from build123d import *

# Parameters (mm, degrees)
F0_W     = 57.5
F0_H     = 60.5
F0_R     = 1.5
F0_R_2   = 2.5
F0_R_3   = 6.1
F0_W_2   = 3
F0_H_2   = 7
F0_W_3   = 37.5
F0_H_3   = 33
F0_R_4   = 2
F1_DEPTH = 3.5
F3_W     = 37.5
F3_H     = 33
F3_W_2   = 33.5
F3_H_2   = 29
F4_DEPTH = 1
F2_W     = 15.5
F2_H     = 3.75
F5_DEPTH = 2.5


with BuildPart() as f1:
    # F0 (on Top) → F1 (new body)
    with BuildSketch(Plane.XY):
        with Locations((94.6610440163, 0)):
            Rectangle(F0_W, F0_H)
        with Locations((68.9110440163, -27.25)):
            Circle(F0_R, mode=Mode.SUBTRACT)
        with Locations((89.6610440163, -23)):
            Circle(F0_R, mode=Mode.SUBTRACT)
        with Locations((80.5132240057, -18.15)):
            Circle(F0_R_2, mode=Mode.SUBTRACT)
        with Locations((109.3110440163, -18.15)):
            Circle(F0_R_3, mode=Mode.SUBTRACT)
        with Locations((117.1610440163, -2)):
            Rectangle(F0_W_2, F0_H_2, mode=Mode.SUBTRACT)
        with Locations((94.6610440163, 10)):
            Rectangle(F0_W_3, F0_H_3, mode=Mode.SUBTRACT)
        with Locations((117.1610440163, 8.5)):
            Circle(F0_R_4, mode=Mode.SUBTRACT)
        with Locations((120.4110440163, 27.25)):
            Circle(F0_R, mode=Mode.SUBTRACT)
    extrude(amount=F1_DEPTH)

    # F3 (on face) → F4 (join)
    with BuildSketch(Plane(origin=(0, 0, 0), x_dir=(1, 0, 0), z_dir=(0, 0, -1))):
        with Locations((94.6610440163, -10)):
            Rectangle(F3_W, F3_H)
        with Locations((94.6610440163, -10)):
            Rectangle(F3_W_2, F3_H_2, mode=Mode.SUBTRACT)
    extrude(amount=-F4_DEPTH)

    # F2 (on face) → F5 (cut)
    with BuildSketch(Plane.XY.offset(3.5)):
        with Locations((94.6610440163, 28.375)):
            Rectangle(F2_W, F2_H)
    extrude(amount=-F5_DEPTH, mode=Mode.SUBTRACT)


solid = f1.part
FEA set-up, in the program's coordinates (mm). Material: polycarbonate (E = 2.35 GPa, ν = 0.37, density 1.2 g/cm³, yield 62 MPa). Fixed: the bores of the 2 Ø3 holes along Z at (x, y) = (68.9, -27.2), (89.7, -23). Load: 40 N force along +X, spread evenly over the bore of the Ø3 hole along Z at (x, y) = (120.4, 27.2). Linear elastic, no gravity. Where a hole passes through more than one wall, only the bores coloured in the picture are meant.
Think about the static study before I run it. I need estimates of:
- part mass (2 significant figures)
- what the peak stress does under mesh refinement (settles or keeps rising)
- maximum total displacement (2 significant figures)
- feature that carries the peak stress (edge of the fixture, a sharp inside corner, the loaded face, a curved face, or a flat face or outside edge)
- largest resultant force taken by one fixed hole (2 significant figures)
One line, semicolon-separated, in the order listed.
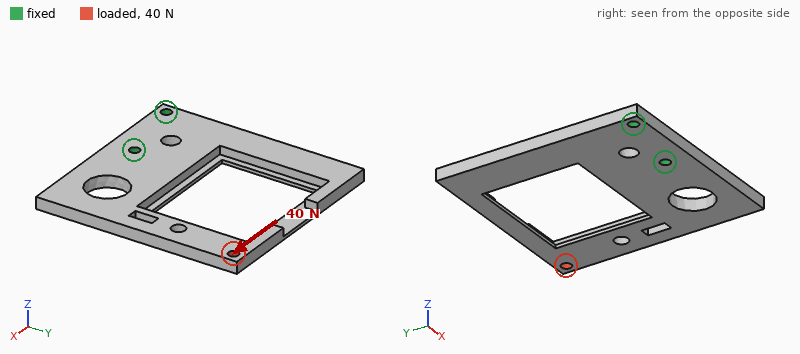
8.8 g; keeps rising; 0.85 mm; a sharp inside corner; 95 N
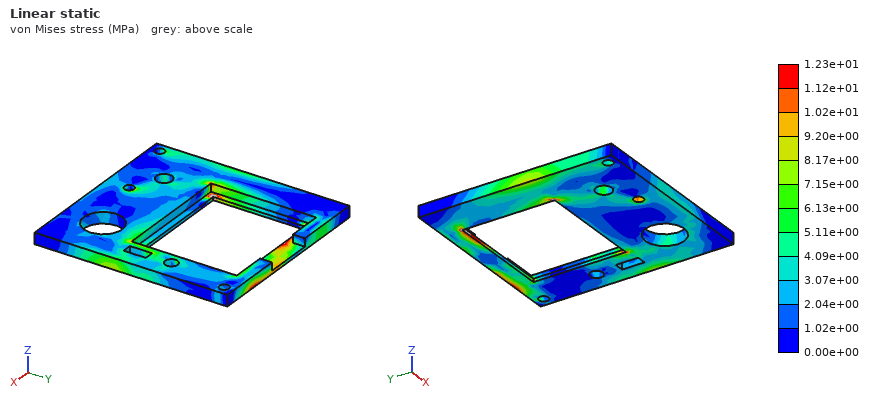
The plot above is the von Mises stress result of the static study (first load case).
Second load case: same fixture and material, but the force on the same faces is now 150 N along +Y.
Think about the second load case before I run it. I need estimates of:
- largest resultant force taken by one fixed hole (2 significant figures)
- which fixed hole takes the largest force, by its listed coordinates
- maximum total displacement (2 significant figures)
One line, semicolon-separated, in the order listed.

350 N; (89.7, -23); 0.92 mm
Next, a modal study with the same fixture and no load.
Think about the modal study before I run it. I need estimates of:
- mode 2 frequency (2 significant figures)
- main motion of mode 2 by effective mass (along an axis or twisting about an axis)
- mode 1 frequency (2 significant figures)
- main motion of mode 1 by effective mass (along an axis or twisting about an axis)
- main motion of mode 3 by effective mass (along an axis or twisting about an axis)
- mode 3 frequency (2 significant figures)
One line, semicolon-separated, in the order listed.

330 Hz; twisting about Y; 230 Hz; along Z; along Z; 660 Hz
